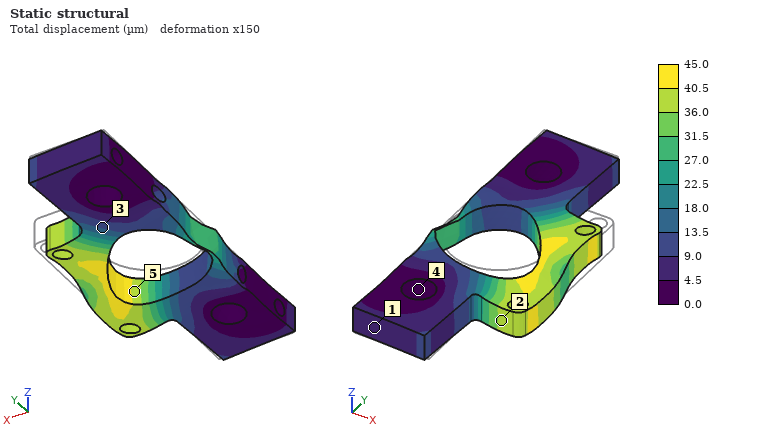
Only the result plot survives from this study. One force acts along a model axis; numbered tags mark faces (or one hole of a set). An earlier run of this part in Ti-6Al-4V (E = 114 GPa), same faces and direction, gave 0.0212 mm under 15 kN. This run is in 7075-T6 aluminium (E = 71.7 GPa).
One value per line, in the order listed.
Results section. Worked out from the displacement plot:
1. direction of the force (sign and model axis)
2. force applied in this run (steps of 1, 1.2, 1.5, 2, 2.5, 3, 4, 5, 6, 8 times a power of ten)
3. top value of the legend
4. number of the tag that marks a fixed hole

-Y
20 kN
45.0 µm
4
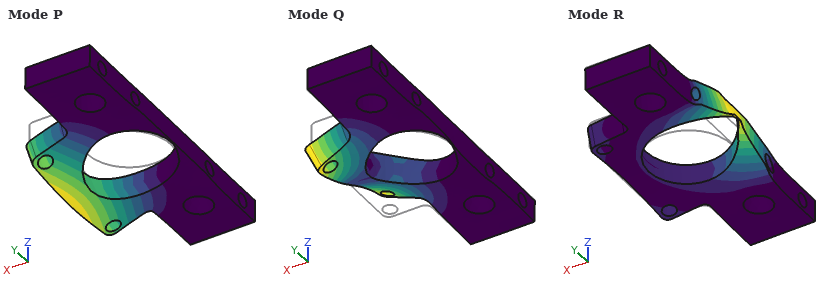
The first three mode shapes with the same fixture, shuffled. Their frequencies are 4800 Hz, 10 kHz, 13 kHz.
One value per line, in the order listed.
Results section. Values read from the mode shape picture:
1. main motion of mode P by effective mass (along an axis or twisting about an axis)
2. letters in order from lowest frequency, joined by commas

along Z
P, Q, R
